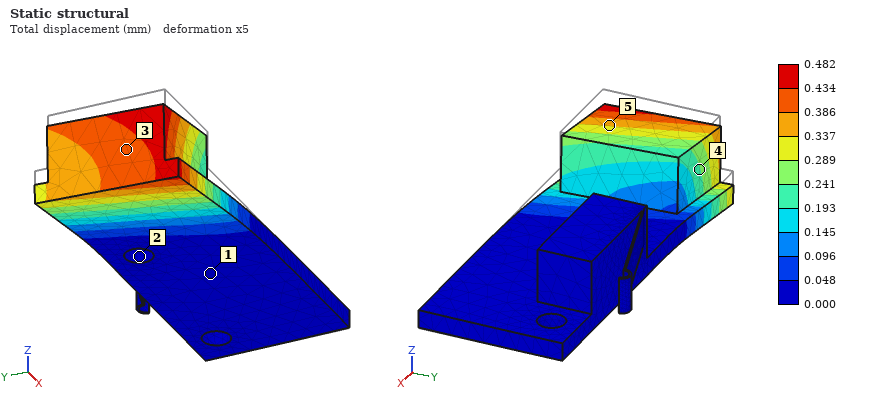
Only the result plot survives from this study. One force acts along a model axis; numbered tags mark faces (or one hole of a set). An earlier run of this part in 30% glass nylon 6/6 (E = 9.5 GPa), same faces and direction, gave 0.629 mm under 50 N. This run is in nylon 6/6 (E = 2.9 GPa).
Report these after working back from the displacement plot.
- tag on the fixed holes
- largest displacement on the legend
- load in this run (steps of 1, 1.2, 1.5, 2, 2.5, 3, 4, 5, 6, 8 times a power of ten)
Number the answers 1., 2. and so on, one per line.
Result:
1. 2
2. 0.482 mm
3. 12 N
